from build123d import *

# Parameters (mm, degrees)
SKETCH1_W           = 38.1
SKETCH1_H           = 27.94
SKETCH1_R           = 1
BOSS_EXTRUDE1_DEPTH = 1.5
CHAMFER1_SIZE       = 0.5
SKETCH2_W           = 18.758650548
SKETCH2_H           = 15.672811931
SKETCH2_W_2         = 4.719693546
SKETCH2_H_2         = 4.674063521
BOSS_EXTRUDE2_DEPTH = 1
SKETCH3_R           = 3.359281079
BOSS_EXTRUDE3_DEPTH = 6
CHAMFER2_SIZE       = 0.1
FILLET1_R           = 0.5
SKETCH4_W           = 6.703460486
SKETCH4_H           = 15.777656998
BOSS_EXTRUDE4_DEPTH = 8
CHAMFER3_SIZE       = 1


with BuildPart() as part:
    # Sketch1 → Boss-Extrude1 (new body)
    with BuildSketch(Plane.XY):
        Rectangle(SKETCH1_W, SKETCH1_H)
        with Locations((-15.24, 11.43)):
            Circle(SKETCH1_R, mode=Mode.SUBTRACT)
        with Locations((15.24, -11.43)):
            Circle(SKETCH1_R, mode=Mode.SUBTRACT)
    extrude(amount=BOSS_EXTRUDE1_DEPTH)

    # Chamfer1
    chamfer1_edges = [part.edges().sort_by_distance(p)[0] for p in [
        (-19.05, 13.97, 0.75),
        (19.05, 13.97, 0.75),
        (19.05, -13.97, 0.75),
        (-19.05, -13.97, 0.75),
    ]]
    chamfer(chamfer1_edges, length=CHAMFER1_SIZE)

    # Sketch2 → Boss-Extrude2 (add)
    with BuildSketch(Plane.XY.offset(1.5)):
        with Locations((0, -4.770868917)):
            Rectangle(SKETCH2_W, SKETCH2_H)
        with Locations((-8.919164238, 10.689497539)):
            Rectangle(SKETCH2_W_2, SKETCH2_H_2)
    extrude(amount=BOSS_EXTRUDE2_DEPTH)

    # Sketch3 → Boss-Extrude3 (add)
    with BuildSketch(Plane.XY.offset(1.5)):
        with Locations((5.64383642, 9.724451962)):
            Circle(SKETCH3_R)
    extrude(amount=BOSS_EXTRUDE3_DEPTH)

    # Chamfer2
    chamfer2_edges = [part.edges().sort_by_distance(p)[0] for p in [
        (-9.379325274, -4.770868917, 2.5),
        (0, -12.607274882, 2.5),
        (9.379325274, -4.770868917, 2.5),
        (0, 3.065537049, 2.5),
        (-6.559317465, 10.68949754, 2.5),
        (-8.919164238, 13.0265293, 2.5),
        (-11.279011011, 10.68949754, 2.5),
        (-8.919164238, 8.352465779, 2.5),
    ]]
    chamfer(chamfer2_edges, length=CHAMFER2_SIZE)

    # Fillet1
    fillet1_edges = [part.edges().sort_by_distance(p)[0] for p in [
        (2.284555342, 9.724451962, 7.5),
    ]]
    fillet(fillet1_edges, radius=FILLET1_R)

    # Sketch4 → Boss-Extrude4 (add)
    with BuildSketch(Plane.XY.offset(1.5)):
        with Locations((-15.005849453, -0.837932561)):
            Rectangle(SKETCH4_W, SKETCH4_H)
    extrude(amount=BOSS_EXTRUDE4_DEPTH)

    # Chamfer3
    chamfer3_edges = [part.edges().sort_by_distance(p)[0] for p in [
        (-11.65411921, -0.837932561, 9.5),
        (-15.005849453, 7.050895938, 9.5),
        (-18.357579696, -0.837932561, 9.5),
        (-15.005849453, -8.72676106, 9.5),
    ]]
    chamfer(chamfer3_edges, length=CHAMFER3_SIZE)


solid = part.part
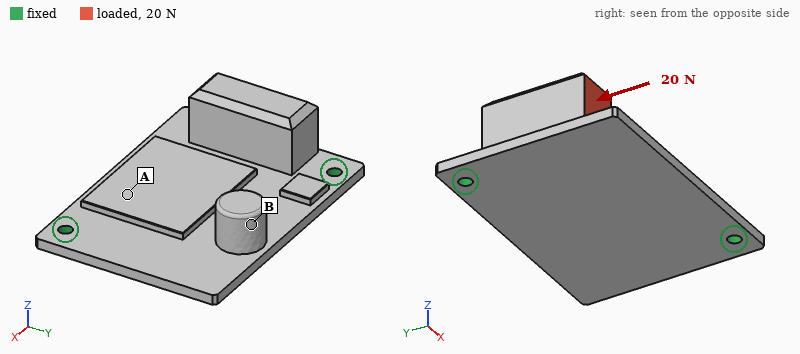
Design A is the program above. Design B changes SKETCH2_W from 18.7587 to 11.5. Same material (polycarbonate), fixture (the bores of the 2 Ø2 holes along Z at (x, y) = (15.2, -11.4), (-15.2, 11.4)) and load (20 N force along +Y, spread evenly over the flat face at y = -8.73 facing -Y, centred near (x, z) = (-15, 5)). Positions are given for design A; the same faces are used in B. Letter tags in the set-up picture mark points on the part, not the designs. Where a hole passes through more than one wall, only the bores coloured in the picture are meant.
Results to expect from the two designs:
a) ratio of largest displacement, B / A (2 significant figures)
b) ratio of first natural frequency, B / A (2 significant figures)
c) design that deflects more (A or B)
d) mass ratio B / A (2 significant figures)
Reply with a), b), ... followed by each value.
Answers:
a) 1.1
b) 0.97
c) B
d) 0.96
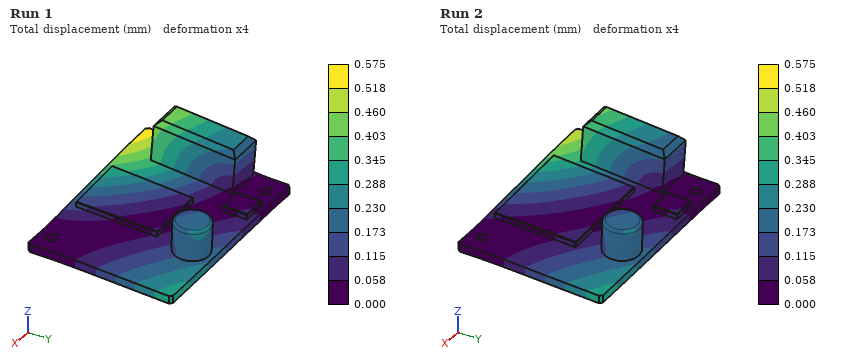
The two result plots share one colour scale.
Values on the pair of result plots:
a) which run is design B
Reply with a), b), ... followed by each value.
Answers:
a) Run 1
